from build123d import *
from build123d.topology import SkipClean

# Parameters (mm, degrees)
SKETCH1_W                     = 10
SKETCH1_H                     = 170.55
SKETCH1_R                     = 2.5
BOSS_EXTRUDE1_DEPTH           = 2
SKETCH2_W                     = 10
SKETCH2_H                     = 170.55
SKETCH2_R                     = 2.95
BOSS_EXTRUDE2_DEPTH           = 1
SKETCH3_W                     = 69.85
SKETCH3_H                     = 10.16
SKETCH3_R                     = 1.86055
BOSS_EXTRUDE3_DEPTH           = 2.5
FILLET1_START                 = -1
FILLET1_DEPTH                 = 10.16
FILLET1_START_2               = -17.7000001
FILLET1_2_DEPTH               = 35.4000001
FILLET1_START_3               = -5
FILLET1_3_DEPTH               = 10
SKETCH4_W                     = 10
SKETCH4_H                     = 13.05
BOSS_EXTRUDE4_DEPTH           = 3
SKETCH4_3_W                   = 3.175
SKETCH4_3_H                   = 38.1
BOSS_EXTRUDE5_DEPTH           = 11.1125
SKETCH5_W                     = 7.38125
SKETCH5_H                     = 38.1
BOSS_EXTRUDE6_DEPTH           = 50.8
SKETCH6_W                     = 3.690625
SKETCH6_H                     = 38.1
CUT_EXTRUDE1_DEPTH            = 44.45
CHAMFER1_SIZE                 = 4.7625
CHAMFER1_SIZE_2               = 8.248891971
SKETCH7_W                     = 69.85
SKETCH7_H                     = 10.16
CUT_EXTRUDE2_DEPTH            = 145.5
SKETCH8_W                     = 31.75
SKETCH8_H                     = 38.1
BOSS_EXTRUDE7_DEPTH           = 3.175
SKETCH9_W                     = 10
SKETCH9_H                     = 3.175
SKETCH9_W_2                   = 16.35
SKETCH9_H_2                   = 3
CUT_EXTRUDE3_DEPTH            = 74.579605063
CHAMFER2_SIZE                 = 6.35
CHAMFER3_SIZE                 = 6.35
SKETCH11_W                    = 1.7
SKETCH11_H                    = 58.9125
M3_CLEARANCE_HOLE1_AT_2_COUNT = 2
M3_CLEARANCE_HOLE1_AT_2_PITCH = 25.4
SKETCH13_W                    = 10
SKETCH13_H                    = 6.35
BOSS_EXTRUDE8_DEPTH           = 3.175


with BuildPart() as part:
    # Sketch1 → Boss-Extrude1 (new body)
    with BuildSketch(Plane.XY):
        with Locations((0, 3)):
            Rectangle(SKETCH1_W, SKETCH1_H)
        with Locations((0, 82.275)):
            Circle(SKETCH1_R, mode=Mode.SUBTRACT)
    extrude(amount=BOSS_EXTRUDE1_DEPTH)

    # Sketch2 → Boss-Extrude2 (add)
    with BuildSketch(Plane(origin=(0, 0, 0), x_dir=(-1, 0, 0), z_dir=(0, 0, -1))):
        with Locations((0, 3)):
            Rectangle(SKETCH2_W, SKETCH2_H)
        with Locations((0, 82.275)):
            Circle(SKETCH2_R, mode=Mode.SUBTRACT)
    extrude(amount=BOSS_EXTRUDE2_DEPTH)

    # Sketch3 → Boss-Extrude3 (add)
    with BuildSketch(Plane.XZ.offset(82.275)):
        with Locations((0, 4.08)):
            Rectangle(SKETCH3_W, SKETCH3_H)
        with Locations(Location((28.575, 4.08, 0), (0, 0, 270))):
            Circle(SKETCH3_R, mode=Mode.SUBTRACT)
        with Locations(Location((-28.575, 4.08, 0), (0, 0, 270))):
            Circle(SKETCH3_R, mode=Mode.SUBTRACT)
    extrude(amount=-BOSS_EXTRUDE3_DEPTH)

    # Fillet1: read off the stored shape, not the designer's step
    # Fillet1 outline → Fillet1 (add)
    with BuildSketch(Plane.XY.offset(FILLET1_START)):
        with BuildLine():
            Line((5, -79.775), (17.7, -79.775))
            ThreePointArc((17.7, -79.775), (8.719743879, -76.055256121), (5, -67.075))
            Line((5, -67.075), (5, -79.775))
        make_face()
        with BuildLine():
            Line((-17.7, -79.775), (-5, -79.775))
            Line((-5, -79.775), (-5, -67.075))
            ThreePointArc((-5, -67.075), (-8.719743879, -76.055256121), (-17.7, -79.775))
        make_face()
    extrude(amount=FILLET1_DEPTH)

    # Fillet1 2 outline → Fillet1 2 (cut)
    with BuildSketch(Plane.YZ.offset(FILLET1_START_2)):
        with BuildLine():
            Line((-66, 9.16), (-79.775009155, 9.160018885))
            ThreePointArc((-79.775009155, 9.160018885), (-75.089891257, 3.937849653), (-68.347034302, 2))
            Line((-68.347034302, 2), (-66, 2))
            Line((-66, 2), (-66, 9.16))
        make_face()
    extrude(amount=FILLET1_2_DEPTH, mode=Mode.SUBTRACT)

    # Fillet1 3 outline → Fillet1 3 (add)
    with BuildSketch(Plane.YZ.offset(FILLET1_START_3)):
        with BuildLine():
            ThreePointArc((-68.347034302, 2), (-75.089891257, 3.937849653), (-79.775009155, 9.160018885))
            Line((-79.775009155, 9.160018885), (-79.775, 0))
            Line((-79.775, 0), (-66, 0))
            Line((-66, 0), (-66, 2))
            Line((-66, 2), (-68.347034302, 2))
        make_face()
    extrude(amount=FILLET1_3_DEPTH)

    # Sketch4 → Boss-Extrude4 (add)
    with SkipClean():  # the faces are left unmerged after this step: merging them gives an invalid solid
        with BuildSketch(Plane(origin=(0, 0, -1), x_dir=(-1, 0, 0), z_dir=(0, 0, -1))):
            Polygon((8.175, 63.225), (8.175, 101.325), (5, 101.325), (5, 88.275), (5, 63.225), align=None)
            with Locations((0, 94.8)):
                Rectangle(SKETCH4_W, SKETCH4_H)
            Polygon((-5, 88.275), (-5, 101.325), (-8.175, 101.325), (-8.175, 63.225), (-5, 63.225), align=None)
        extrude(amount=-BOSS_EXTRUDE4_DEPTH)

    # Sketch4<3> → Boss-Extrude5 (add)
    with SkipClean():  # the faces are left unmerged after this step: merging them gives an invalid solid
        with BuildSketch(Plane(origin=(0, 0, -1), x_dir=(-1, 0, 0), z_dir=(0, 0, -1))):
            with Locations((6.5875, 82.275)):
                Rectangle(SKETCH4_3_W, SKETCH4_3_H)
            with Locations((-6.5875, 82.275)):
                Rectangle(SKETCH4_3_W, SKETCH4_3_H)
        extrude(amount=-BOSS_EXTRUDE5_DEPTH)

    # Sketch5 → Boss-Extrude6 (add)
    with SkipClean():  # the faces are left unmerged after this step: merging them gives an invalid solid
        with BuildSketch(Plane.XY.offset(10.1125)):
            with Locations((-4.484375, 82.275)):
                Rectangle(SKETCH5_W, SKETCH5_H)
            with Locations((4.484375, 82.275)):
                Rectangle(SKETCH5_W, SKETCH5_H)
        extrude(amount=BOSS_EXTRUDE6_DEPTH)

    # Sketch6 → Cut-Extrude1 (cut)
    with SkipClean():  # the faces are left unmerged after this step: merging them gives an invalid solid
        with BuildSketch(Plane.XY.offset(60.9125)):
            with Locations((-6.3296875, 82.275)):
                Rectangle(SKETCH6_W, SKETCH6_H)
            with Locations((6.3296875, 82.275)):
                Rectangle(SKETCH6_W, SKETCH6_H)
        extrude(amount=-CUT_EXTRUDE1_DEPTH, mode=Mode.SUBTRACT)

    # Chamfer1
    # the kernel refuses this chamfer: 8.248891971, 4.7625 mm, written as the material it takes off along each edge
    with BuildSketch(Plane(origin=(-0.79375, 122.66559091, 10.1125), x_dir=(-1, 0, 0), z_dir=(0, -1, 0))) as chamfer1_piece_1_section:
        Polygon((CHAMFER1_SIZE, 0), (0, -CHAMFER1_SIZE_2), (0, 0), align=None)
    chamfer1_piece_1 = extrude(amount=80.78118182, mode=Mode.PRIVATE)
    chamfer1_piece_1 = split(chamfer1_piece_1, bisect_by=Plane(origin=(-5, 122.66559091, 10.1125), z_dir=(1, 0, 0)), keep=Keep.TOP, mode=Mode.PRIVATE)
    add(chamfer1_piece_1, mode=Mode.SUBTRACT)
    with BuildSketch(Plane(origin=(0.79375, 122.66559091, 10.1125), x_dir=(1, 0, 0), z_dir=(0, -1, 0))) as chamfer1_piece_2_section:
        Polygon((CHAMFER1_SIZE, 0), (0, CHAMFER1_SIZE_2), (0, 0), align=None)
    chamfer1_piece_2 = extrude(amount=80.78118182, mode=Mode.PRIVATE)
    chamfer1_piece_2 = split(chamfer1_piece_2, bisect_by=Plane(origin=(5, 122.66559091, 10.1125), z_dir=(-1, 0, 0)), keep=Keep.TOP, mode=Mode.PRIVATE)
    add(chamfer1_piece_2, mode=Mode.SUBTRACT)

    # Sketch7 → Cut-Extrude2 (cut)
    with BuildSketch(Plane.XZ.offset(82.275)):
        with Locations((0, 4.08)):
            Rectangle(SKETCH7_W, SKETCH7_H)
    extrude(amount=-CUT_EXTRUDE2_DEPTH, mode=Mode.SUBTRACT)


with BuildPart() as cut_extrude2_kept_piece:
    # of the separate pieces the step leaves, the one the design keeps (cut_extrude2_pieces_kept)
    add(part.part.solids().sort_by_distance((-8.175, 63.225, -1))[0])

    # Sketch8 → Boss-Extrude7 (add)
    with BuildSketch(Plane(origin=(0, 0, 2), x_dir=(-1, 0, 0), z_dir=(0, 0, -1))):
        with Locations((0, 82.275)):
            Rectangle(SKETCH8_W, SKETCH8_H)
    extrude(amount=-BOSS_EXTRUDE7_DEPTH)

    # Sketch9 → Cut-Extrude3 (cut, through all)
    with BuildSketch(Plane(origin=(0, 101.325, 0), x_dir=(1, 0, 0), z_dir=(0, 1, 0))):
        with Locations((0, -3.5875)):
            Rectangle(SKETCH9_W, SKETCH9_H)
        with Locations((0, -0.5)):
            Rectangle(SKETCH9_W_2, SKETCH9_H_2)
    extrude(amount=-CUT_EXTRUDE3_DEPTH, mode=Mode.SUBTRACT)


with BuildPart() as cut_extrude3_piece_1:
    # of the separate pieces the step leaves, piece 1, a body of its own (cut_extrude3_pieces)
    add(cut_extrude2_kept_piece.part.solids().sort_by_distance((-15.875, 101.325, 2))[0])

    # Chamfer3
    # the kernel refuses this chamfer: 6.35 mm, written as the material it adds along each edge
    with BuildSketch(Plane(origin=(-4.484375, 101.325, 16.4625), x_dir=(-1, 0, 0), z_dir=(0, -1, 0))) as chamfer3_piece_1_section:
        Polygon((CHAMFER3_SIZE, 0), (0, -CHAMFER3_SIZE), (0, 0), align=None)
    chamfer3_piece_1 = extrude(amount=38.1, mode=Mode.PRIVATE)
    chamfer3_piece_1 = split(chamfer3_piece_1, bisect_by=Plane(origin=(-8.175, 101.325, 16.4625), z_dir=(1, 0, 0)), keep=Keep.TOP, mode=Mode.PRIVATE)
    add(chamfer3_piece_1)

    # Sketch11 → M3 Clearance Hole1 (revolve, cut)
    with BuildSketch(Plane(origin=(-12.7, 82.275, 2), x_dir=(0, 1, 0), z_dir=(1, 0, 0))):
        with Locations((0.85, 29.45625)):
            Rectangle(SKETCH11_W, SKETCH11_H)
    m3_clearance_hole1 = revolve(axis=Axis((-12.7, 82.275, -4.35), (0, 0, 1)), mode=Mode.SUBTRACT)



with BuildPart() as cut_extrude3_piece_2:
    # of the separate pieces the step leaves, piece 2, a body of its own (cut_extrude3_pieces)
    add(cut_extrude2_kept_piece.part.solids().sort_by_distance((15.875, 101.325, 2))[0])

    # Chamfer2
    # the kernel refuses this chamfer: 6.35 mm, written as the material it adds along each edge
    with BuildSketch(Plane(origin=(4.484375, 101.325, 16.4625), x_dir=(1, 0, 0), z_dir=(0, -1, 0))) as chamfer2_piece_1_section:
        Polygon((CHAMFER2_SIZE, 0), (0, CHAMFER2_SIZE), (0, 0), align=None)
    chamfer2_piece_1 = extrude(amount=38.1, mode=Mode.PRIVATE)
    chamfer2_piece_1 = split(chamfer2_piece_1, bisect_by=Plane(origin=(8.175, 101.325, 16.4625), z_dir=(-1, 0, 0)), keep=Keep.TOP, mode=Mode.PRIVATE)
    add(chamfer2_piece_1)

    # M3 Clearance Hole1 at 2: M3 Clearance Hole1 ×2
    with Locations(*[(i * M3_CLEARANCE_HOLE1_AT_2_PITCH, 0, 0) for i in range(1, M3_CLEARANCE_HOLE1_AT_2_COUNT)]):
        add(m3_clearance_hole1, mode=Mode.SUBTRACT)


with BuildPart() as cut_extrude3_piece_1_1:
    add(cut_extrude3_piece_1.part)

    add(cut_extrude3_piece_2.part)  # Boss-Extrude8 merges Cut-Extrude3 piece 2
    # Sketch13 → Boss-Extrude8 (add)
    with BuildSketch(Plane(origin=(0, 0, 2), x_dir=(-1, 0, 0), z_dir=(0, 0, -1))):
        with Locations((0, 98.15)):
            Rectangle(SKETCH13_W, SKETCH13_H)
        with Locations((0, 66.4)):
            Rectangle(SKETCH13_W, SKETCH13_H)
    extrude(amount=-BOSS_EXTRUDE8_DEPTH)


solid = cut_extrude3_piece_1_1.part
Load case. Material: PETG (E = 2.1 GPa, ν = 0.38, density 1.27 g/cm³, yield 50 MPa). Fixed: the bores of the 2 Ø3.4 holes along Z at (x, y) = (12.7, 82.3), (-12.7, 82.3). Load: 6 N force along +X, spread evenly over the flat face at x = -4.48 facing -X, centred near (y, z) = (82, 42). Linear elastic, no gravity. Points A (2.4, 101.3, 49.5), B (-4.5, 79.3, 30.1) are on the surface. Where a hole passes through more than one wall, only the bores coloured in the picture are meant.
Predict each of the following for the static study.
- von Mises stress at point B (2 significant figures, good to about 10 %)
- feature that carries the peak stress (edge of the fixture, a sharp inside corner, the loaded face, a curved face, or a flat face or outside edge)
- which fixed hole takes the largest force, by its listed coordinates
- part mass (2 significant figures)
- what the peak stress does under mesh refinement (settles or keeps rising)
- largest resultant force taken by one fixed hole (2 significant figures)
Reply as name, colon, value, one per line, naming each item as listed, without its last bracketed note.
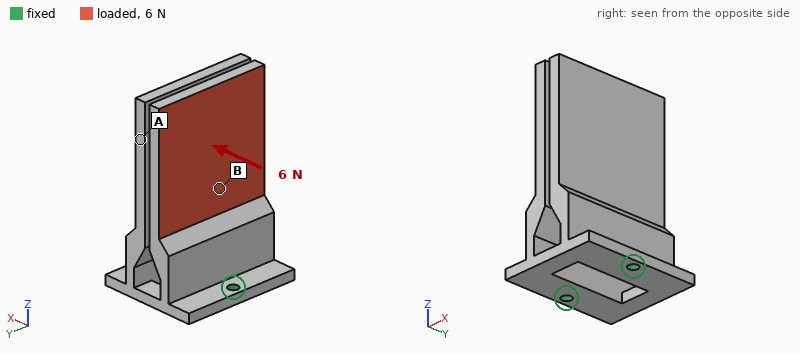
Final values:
von Mises stress at point B: 0.85 MPa
feature that carries the peak stress: edge of the fixture
which fixed hole takes the largest force, by its listed coordinates: (-12.7, 82.3)
part mass: 25 g
what the peak stress does under mesh refinement: keeps rising
largest resultant force taken by one fixed hole: 9.9 N
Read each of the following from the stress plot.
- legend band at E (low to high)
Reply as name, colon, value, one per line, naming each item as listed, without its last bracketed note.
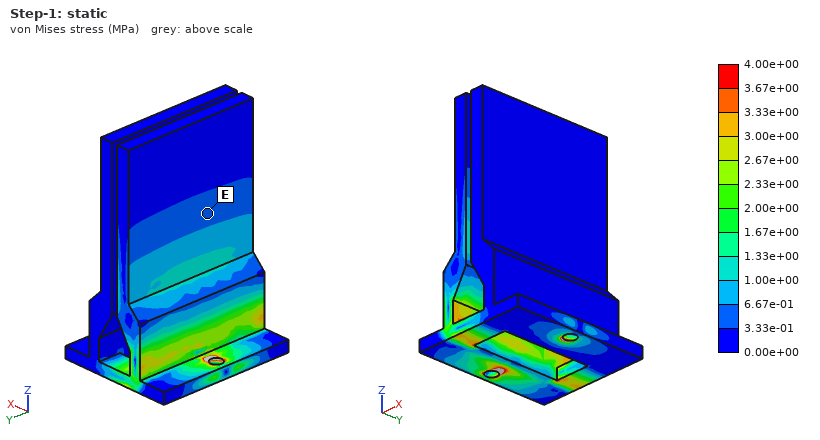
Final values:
legend band at E: 3.33e-01 to 6.67e-01 MPa
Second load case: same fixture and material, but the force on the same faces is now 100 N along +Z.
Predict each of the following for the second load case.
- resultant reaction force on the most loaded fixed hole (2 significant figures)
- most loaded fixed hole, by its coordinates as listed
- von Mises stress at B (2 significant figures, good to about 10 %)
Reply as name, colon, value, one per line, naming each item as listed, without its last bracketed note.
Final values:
resultant reaction force on the most loaded fixed hole: 78 N
most loaded fixed hole, by its coordinates as listed: (-12.7, 82.3)
von Mises stress at B: 2.2 MPa
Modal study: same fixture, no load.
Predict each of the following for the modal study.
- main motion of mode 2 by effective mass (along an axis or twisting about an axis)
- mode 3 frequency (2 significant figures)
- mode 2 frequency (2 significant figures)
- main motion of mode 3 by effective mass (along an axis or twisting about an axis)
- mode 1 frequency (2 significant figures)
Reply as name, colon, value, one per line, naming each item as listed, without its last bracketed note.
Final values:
main motion of mode 2 by effective mass: along X
mode 3 frequency: 250 Hz
mode 2 frequency: 210 Hz
main motion of mode 3 by effective mass: along Y
mode 1 frequency: 180 Hz
